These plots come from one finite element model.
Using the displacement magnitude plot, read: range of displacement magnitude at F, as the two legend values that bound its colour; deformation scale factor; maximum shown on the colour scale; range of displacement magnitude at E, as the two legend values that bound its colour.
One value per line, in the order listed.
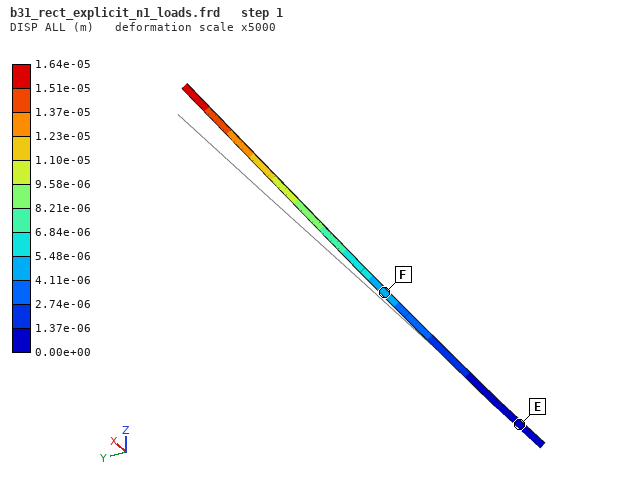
4.11e-06 to 5.48e-06 m
5000
1.64e-05 m
0.00e+00 to 1.37e-06 m
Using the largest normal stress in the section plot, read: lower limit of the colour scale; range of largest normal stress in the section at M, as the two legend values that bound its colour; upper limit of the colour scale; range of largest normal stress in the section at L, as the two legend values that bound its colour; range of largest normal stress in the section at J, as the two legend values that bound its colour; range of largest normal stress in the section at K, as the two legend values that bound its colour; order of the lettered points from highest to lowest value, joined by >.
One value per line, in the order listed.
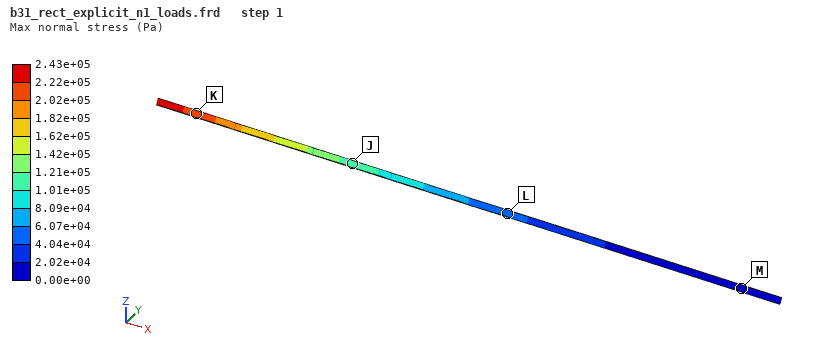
0.00e+00 Pa
0.00e+00 to 2.02e+04 Pa
2.43e+05 Pa
4.04e+04 to 6.07e+04 Pa
1.01e+05 to 1.21e+05 Pa
2.02e+05 to 2.22e+05 Pa
K > J > L > M
